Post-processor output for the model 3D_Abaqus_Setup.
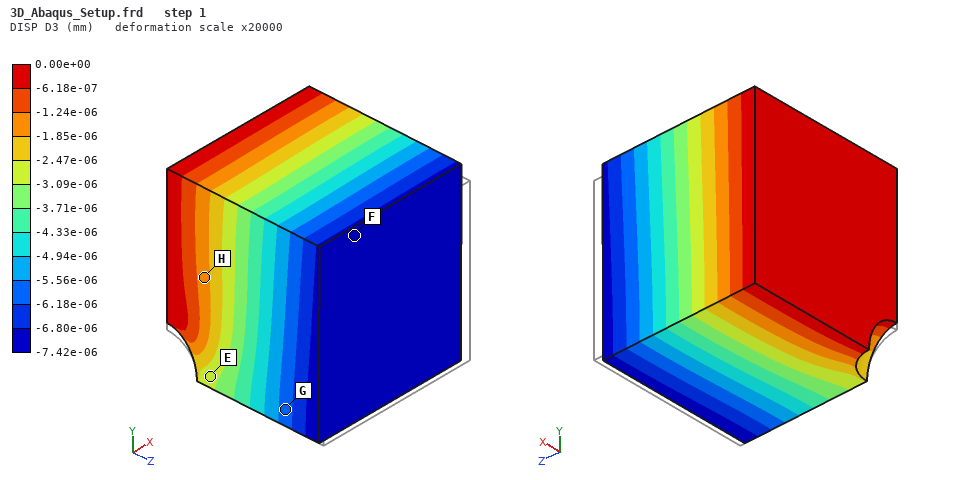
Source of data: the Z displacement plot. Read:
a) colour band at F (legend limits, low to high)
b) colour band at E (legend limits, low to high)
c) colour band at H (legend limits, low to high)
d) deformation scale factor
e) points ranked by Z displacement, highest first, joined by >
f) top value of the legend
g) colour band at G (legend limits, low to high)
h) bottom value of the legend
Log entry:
-7.42e-06 to -6.80e-06 mm
-3.09e-06 to -2.47e-06 mm
-1.85e-06 to -1.24e-06 mm
20000
H > E > G > F
0.00e+00 mm
-6.18e-06 to -5.56e-06 mm
-7.42e-06 mm
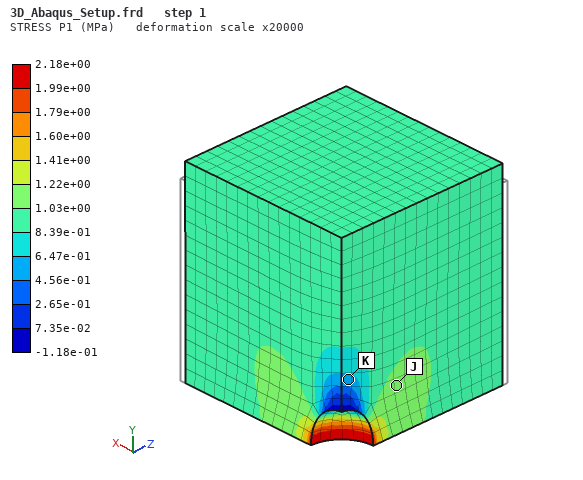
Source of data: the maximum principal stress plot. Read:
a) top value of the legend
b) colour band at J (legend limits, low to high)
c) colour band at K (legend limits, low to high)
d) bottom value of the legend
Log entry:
2.18e+00 MPa
1.03e+00 to 1.22e+00 MPa
4.56e-01 to 6.47e-01 MPa
-1.18e-01 MPa
